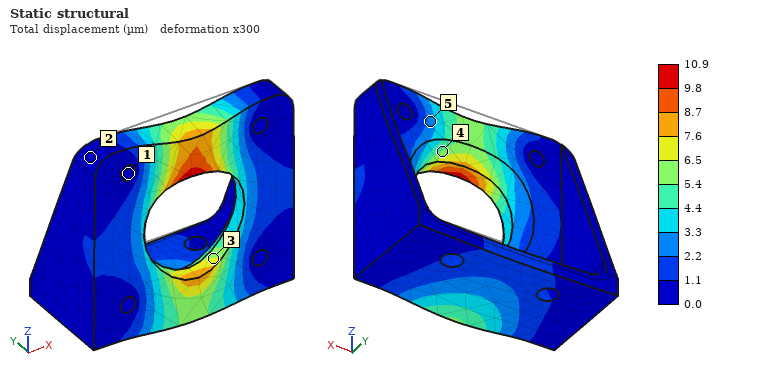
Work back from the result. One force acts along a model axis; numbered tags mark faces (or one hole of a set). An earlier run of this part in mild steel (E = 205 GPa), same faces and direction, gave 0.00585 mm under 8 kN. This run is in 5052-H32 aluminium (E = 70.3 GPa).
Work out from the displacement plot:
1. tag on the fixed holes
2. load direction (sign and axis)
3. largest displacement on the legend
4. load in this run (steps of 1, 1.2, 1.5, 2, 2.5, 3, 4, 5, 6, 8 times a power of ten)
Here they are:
1
-Z
10.9 µm
5 kN
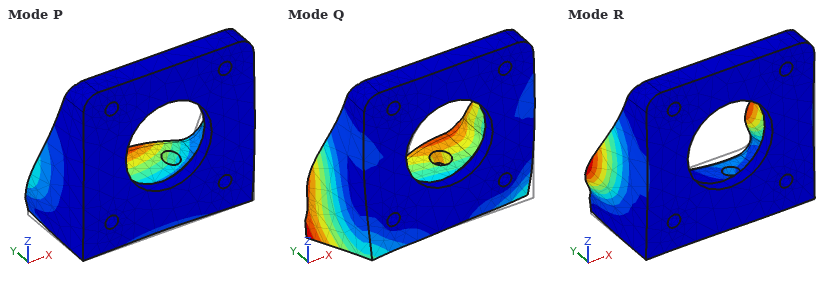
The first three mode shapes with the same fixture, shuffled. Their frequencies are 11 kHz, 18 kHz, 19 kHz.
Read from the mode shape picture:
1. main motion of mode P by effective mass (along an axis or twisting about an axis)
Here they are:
along Z
